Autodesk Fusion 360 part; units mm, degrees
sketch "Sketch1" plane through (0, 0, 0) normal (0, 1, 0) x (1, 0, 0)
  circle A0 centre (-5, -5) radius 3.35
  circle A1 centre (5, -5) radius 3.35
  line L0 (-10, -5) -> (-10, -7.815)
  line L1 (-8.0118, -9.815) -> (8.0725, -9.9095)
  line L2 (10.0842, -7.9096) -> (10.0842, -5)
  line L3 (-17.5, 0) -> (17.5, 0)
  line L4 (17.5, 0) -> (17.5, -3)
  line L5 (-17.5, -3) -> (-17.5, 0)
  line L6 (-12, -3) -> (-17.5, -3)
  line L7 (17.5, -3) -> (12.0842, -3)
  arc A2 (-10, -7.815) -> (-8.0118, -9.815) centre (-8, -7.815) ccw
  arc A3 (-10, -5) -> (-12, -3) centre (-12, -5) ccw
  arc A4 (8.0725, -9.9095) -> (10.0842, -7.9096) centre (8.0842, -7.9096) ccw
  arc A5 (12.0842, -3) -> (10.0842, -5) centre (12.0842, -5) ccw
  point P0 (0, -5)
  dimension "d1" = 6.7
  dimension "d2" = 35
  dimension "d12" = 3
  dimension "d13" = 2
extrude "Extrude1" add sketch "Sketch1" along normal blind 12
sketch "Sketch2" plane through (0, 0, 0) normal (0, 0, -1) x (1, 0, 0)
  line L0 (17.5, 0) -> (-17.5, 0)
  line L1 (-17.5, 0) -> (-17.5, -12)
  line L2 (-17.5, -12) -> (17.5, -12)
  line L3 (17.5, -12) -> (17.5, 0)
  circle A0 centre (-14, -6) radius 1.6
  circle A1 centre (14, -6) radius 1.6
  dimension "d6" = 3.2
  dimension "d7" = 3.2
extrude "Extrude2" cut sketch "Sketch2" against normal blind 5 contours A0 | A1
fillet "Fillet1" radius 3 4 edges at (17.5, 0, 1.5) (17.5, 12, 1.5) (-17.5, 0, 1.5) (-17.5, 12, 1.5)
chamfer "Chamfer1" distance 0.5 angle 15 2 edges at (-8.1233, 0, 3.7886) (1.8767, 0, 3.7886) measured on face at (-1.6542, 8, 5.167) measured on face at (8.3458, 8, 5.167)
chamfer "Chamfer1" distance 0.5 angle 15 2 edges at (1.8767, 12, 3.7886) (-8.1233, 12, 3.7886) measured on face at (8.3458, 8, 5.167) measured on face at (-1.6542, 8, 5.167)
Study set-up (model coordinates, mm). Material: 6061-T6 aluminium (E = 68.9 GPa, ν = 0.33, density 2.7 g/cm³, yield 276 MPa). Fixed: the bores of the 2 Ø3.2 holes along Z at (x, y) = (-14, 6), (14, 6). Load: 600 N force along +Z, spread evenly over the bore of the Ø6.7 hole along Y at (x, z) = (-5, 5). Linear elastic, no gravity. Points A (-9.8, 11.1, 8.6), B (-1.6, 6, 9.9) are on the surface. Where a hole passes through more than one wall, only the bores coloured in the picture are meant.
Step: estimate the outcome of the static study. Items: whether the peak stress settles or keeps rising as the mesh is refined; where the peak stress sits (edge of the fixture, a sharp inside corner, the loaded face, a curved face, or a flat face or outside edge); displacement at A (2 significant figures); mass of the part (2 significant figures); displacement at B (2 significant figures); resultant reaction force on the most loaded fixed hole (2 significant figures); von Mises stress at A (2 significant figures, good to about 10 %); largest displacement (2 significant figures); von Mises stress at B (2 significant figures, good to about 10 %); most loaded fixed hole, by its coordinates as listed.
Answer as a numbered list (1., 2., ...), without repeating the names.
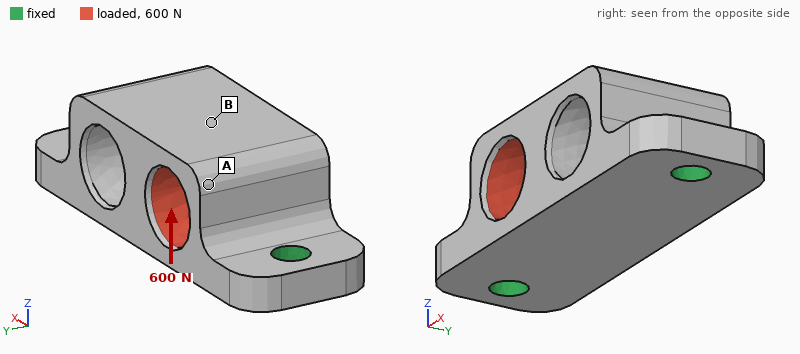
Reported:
1. keeps rising
2. edge of the fixture
3. 6.2 µm
4. 5.4 g
5. 9.6 µm
6. 440 N
7. 7.4 MPa
8. 10 µm
9. 24 MPa
10. (-14, 6)
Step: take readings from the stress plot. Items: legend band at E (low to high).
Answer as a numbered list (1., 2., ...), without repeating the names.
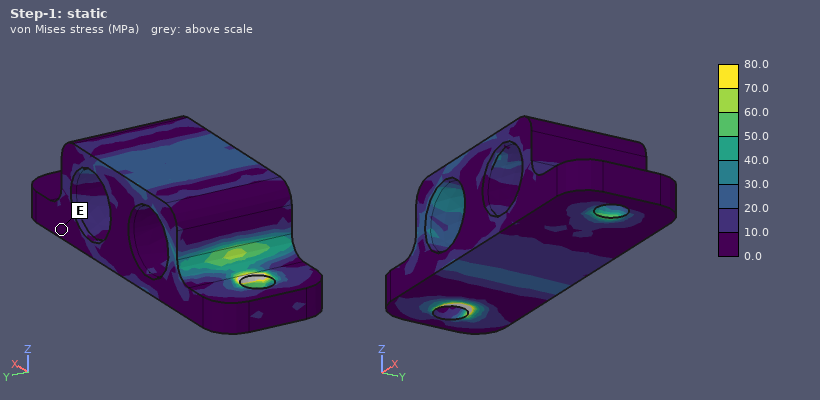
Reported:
1. 0.0 to 10.0 MPa
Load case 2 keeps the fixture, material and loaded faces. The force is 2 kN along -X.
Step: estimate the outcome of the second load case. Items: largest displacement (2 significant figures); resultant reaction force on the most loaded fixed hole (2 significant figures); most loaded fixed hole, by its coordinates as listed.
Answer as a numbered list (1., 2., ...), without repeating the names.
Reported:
1. 14 µm
2. 1.3 kN
3. (-14, 6)
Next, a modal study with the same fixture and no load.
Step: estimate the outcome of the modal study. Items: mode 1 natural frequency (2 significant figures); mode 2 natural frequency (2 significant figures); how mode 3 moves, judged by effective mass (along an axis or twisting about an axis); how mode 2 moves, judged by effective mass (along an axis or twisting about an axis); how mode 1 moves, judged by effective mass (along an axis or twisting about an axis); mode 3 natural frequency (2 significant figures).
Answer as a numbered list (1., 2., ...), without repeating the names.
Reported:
1. 16 kHz
2. 22 kHz
3. along Y
4. along Z
5. along Y
6. 32 kHz
